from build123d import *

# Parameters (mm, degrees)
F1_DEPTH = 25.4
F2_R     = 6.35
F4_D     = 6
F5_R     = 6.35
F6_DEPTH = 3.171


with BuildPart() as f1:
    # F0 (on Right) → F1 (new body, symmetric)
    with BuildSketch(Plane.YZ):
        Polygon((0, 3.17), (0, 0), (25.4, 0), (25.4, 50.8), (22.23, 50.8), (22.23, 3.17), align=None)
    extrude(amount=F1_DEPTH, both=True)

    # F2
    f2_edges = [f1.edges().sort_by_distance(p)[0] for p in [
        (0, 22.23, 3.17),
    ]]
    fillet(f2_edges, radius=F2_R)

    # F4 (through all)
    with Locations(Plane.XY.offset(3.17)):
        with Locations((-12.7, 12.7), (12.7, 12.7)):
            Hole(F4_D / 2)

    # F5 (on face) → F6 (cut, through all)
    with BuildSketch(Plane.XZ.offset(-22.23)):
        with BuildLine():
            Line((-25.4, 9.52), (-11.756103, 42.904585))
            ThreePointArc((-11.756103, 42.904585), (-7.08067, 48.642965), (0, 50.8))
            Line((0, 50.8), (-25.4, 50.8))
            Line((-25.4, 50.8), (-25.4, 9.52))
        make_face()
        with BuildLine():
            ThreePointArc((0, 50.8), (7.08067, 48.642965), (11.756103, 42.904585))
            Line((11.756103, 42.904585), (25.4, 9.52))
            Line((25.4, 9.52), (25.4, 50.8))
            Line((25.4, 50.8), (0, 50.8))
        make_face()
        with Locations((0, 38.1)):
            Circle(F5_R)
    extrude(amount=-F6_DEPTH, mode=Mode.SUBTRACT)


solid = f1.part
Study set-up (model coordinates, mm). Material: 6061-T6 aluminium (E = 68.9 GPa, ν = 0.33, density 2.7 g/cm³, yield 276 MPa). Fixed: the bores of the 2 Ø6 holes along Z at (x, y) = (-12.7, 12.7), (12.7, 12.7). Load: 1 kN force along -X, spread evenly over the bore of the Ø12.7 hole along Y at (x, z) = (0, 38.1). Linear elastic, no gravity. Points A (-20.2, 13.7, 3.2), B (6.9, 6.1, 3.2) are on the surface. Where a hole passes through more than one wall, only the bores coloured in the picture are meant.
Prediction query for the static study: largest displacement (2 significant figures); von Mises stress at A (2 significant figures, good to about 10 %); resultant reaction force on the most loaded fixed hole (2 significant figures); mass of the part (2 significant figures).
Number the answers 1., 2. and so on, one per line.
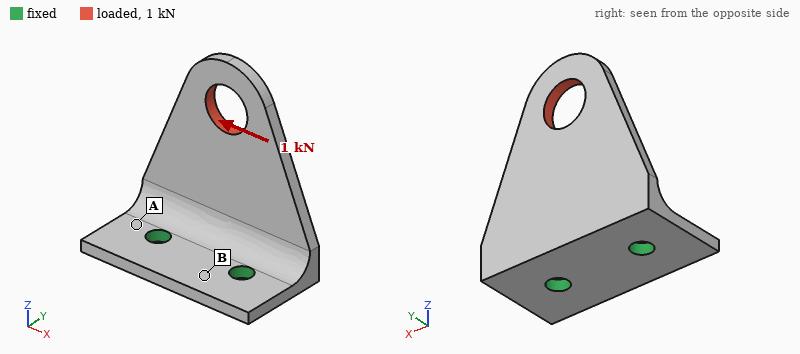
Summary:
1. 0.19 mm
2. 75 MPa
3. 1.4 kN
4. 25 g
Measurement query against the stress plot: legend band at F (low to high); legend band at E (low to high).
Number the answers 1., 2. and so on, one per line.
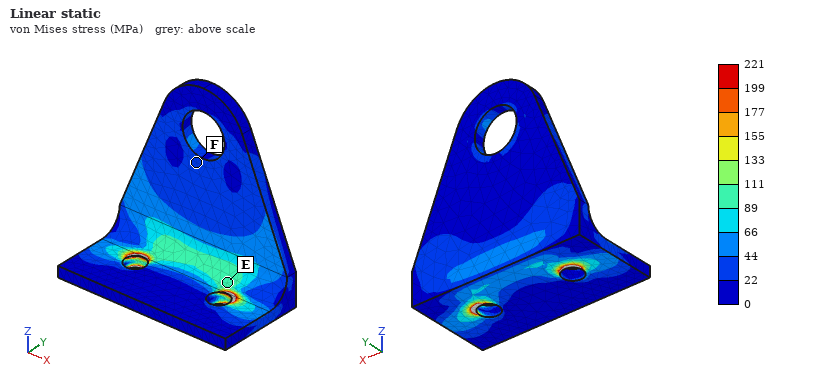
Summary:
1. 22 to 44 MPa
2. 89 to 111 MPa
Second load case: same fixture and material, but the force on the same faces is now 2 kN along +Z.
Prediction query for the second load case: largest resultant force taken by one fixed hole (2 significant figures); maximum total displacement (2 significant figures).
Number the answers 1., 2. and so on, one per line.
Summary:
1. 1.0 kN
2. 0.44 mm
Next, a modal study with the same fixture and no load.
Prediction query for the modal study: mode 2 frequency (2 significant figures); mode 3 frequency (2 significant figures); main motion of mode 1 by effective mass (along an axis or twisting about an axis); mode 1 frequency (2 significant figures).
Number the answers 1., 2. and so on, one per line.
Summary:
1. 4300 Hz
2. 5700 Hz
3. along Y
4. 1600 Hz
